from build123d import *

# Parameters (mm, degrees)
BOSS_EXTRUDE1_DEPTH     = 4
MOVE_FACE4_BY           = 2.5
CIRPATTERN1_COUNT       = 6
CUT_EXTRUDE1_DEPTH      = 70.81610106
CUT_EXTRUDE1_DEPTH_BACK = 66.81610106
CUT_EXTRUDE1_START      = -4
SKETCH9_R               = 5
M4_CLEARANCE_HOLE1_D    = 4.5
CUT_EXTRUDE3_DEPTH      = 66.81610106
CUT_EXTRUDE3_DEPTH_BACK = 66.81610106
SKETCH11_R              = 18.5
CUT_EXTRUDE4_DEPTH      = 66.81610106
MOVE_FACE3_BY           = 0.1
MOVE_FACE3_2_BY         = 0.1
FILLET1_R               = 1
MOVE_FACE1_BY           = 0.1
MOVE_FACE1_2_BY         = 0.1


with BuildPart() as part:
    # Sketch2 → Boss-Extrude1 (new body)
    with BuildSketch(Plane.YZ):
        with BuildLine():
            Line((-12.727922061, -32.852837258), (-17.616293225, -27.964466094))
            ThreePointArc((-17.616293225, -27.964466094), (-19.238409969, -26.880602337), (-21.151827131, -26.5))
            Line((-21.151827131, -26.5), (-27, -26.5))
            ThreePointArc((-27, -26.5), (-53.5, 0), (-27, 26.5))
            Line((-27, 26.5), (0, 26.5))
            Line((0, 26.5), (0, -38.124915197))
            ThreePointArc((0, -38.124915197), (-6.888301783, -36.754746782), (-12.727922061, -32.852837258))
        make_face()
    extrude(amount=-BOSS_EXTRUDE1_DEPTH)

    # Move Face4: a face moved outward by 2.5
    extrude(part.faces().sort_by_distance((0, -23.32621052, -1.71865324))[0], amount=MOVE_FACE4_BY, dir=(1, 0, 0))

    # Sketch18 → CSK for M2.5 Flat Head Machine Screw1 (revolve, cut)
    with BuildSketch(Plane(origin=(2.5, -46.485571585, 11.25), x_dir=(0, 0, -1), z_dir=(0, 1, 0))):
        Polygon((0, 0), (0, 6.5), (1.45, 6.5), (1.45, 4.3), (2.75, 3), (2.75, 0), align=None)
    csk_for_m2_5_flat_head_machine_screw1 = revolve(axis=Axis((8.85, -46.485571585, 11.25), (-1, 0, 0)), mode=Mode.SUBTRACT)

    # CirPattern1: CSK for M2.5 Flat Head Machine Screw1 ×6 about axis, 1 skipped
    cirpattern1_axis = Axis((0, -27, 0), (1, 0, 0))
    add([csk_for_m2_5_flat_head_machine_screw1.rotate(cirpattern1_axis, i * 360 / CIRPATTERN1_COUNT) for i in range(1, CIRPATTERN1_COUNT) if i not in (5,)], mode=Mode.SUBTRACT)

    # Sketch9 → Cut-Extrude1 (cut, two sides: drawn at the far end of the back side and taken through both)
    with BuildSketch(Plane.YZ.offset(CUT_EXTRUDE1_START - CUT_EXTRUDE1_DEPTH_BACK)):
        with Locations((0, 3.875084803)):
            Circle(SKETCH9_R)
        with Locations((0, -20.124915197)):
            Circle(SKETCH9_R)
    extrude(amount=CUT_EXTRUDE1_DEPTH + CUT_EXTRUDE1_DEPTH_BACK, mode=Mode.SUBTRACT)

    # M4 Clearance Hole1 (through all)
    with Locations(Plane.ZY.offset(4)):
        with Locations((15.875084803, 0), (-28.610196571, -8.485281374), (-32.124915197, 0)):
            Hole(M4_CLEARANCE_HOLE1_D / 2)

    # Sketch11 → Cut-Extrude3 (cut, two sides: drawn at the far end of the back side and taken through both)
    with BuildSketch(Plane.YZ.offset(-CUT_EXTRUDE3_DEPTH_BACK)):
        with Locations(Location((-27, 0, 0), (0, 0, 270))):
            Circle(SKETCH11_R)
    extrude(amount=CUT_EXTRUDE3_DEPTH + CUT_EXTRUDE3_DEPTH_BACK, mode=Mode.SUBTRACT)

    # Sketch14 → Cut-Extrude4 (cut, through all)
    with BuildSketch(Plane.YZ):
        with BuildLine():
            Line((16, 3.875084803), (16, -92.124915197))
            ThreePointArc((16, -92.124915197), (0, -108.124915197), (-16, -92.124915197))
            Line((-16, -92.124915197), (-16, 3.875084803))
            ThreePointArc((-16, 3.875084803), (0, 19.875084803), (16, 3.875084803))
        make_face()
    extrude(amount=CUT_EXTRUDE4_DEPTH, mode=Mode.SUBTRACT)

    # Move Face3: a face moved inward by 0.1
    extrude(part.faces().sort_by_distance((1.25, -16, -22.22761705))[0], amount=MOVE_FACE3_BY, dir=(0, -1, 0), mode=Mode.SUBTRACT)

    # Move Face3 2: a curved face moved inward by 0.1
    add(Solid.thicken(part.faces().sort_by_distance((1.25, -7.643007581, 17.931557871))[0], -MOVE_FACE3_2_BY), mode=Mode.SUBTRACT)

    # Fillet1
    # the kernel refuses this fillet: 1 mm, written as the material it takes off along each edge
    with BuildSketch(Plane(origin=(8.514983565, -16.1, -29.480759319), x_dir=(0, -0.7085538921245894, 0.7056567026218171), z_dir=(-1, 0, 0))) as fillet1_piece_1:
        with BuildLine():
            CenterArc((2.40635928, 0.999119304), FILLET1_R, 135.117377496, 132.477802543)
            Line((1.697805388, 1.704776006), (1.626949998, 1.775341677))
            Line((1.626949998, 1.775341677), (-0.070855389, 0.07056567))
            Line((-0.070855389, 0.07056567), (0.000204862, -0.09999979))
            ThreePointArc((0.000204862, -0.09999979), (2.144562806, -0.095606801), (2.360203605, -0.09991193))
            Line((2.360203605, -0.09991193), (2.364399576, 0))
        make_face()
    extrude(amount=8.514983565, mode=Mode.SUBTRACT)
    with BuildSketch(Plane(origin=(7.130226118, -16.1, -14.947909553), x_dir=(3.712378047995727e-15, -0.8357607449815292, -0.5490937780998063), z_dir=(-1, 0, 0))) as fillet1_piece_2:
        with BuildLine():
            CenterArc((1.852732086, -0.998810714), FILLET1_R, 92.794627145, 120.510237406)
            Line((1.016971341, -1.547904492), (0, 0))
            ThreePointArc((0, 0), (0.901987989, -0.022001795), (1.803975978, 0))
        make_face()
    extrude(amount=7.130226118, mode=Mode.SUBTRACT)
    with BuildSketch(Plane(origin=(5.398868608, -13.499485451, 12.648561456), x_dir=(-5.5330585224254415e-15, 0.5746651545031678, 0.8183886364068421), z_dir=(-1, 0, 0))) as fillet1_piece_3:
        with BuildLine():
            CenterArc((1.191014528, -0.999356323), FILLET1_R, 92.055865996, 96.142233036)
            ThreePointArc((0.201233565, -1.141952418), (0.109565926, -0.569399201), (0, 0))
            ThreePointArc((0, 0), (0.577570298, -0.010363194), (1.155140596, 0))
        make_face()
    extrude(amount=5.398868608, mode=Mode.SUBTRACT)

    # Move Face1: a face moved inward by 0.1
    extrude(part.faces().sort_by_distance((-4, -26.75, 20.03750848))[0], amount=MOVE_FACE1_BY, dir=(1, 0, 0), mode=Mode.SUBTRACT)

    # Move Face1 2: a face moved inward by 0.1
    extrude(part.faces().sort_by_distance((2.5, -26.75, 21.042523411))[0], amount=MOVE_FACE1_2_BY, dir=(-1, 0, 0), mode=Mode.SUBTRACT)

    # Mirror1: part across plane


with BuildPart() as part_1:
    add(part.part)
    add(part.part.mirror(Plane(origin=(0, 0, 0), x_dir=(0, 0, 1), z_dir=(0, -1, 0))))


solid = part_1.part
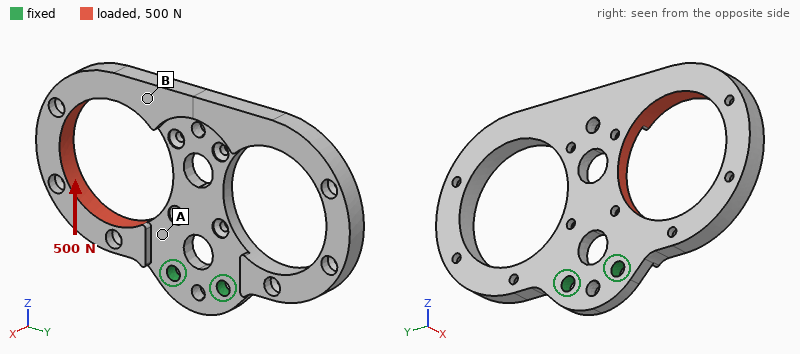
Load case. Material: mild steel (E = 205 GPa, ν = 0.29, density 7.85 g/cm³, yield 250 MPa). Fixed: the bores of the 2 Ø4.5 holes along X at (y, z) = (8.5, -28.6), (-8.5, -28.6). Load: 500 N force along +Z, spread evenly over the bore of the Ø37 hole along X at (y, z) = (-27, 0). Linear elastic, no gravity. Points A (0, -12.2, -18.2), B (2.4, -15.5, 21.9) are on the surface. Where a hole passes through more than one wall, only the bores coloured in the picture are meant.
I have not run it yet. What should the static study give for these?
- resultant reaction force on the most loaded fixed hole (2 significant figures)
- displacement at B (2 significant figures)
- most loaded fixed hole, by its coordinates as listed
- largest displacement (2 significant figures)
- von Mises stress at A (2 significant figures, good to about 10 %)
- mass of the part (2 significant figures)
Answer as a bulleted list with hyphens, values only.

- 870 N
- 21 µm
- (-8.5, -28.6)
- 30 µm
- 18 MPa
- 120 g
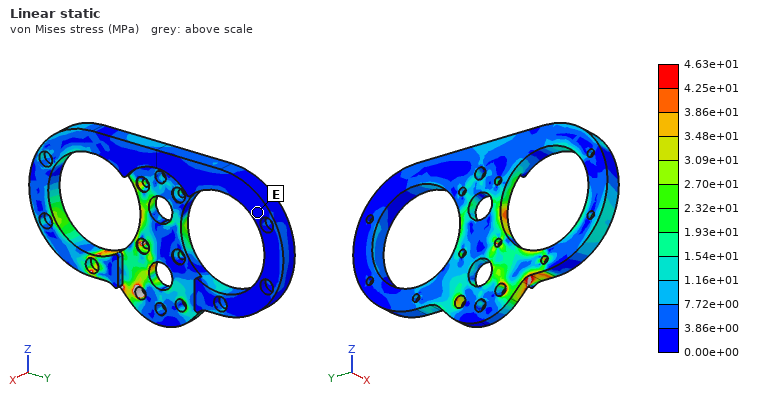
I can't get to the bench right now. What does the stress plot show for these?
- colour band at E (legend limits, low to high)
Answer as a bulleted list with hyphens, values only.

- 0.00e+00 to 3.86e+00 MPa
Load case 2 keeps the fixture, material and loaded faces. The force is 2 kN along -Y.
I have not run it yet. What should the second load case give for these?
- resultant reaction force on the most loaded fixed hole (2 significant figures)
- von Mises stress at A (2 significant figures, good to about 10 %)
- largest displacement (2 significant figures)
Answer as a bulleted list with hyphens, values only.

- 2.7 kN
- 65 MPa
- 94 µm
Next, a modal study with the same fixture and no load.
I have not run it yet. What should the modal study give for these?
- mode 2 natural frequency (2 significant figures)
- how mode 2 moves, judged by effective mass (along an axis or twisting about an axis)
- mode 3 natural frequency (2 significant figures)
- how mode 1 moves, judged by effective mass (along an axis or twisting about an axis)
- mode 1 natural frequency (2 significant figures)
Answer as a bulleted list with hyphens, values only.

- 900 Hz
- twisting about Z
- 2000 Hz
- along X
- 640 Hz
